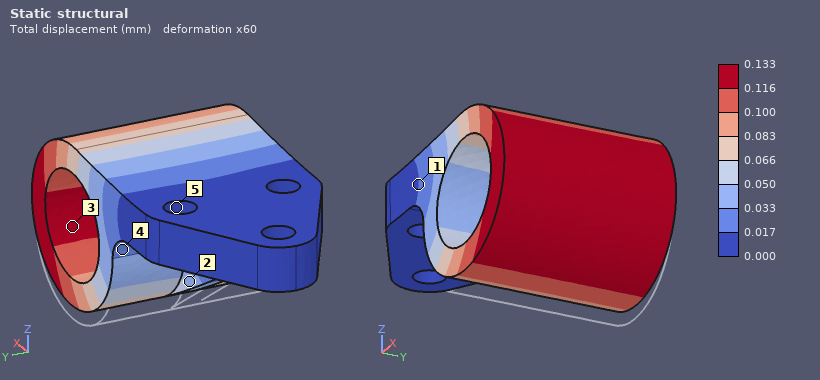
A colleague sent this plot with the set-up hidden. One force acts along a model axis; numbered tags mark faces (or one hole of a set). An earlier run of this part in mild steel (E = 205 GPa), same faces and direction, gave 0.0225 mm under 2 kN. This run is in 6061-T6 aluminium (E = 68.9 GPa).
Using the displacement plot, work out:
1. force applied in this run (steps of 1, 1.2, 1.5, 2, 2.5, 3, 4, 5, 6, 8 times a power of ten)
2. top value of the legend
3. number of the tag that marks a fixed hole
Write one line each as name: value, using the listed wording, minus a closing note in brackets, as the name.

force applied in this run: 4 kN
top value of the legend: 0.133 mm
number of the tag that marks a fixed hole: 5
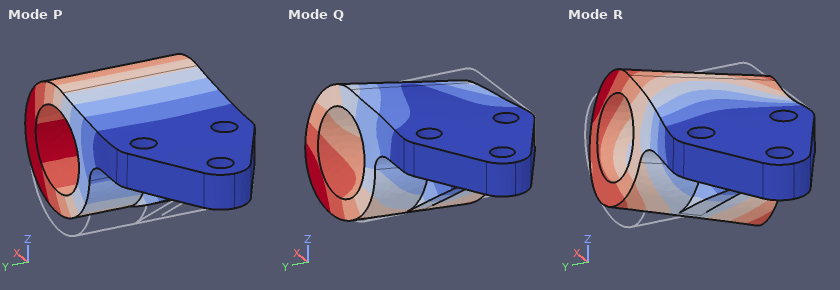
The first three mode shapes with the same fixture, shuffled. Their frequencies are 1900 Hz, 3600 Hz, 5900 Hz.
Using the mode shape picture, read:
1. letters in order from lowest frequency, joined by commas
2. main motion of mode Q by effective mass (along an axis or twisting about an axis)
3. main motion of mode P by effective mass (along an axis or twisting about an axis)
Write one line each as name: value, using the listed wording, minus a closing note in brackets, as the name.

letters in order from lowest frequency, joined by commas: P, Q, R
main motion of mode Q by effective mass: along Y
main motion of mode P by effective mass: along Z
